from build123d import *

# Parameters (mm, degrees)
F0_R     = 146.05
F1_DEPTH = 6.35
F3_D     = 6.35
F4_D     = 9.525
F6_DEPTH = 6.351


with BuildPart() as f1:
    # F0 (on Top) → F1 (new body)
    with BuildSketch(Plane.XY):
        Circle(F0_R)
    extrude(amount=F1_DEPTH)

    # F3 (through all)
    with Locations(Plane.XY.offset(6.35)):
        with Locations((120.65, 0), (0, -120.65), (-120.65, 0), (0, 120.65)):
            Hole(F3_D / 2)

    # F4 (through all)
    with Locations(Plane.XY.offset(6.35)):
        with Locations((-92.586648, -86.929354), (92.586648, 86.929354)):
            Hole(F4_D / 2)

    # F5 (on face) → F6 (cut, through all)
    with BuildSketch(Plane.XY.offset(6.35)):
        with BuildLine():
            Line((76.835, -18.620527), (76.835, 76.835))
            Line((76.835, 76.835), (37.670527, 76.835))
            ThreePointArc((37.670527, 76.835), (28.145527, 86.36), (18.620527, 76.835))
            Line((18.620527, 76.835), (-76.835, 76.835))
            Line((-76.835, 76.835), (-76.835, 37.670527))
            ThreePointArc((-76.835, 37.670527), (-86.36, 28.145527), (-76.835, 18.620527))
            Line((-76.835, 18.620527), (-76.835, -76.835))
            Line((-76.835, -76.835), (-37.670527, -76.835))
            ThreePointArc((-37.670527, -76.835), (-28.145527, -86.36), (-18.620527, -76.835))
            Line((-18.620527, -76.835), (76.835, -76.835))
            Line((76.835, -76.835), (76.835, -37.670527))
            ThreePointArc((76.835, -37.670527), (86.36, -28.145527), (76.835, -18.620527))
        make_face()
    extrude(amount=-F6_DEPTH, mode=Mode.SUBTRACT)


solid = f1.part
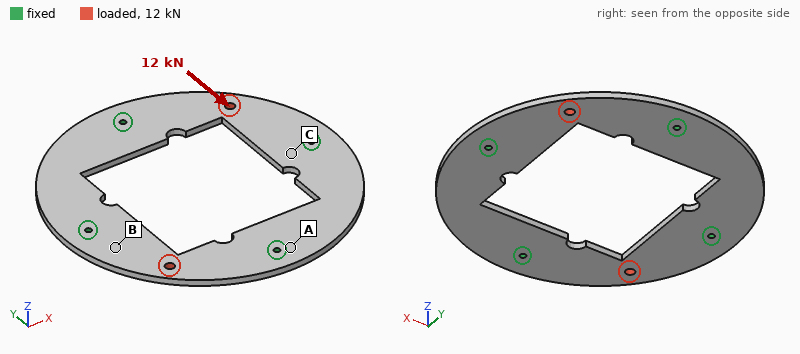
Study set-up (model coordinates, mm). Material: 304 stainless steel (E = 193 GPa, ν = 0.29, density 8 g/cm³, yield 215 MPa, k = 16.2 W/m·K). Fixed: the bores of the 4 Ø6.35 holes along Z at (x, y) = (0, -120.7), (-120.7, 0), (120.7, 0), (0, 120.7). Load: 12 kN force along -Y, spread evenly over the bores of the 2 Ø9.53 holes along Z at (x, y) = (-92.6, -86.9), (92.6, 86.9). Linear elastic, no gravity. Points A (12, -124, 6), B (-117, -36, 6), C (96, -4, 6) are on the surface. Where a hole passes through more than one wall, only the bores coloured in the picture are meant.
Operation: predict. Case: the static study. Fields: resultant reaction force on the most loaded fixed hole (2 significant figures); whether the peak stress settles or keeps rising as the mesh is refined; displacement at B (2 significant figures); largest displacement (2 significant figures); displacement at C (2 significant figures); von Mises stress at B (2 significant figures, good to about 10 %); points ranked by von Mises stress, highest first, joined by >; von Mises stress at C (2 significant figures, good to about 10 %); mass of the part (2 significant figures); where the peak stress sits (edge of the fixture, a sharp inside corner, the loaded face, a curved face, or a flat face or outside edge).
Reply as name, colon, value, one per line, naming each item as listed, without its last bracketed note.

resultant reaction force on the most loaded fixed hole: 5.0 kN
whether the peak stress settles or keeps rising as the mesh is refined: keeps rising
displacement at B: 4.4 µm
largest displacement: 14 µm
displacement at C: 3.6 µm
von Mises stress at B: 16 MPa
points ranked by von Mises stress, highest first, joined by >: B > C > A
von Mises stress at C: 9.9 MPa
mass of the part: 2.2 kg
where the peak stress sits: edge of the fixture
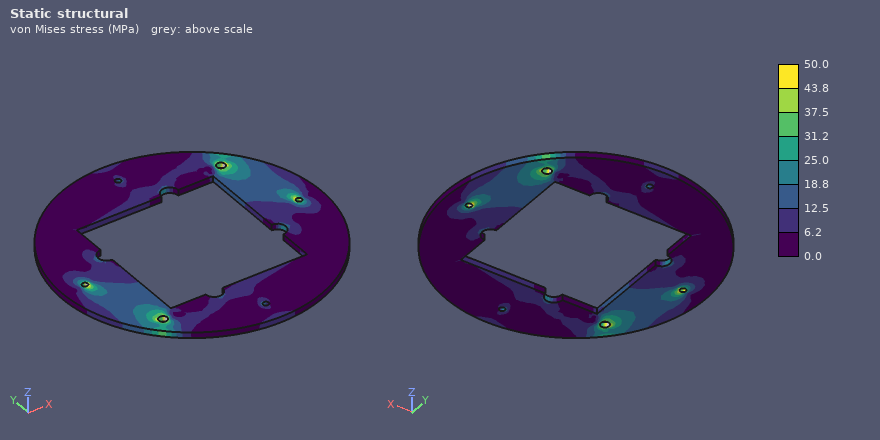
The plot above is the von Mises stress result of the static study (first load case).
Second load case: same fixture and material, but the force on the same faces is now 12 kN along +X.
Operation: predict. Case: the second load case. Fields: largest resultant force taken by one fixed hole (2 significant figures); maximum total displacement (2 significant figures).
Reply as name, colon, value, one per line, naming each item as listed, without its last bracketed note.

largest resultant force taken by one fixed hole: 4.7 kN
maximum total displacement: 15 µm
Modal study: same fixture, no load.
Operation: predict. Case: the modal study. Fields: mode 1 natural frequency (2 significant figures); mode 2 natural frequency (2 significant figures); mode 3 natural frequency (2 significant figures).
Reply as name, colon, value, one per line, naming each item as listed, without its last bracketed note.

mode 1 natural frequency: 700 Hz
mode 2 natural frequency: 780 Hz
mode 3 natural frequency: 780 Hz
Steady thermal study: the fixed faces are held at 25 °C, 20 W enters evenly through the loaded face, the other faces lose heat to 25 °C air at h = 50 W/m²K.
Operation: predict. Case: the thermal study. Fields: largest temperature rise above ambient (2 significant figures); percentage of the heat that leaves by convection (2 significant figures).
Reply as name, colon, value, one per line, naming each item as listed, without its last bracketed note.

largest temperature rise above ambient: 42 K
percentage of the heat that leaves by convection: 94 %
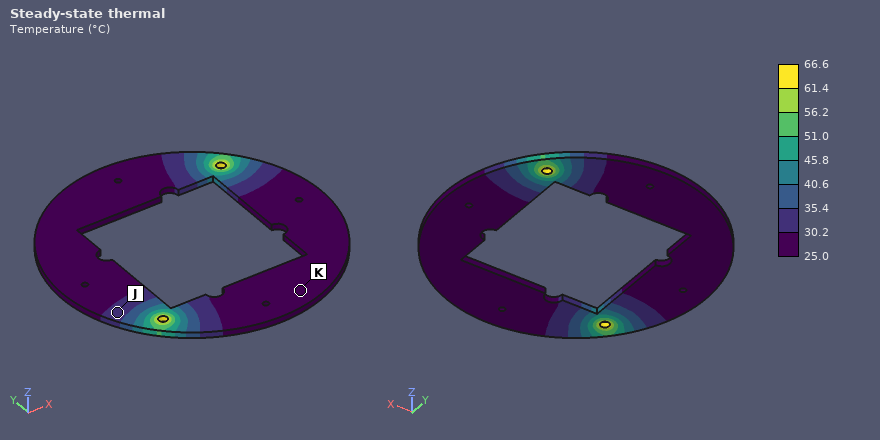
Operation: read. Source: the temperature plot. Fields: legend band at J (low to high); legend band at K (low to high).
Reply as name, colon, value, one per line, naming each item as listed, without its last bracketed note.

legend band at J: 30.2 to 35.4 °C
legend band at K: 25.0 to 30.2 °C
